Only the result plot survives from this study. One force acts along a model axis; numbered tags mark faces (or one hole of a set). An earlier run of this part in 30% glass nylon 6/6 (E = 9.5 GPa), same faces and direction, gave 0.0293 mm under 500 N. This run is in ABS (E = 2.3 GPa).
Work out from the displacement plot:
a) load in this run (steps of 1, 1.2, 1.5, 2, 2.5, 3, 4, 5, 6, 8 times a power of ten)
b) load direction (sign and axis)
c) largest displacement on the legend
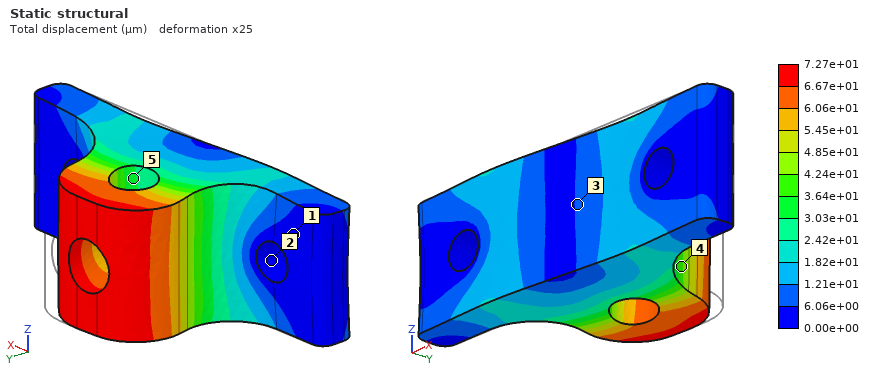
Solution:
300 N
-X
7.27e+01 µm
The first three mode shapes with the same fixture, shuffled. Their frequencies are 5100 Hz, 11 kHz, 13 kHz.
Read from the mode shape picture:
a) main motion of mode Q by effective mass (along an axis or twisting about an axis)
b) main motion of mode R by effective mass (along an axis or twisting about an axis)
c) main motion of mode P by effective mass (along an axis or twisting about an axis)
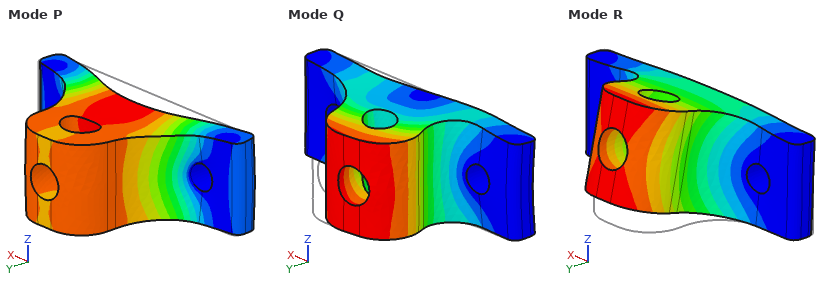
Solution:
along X
along Z
along Y
